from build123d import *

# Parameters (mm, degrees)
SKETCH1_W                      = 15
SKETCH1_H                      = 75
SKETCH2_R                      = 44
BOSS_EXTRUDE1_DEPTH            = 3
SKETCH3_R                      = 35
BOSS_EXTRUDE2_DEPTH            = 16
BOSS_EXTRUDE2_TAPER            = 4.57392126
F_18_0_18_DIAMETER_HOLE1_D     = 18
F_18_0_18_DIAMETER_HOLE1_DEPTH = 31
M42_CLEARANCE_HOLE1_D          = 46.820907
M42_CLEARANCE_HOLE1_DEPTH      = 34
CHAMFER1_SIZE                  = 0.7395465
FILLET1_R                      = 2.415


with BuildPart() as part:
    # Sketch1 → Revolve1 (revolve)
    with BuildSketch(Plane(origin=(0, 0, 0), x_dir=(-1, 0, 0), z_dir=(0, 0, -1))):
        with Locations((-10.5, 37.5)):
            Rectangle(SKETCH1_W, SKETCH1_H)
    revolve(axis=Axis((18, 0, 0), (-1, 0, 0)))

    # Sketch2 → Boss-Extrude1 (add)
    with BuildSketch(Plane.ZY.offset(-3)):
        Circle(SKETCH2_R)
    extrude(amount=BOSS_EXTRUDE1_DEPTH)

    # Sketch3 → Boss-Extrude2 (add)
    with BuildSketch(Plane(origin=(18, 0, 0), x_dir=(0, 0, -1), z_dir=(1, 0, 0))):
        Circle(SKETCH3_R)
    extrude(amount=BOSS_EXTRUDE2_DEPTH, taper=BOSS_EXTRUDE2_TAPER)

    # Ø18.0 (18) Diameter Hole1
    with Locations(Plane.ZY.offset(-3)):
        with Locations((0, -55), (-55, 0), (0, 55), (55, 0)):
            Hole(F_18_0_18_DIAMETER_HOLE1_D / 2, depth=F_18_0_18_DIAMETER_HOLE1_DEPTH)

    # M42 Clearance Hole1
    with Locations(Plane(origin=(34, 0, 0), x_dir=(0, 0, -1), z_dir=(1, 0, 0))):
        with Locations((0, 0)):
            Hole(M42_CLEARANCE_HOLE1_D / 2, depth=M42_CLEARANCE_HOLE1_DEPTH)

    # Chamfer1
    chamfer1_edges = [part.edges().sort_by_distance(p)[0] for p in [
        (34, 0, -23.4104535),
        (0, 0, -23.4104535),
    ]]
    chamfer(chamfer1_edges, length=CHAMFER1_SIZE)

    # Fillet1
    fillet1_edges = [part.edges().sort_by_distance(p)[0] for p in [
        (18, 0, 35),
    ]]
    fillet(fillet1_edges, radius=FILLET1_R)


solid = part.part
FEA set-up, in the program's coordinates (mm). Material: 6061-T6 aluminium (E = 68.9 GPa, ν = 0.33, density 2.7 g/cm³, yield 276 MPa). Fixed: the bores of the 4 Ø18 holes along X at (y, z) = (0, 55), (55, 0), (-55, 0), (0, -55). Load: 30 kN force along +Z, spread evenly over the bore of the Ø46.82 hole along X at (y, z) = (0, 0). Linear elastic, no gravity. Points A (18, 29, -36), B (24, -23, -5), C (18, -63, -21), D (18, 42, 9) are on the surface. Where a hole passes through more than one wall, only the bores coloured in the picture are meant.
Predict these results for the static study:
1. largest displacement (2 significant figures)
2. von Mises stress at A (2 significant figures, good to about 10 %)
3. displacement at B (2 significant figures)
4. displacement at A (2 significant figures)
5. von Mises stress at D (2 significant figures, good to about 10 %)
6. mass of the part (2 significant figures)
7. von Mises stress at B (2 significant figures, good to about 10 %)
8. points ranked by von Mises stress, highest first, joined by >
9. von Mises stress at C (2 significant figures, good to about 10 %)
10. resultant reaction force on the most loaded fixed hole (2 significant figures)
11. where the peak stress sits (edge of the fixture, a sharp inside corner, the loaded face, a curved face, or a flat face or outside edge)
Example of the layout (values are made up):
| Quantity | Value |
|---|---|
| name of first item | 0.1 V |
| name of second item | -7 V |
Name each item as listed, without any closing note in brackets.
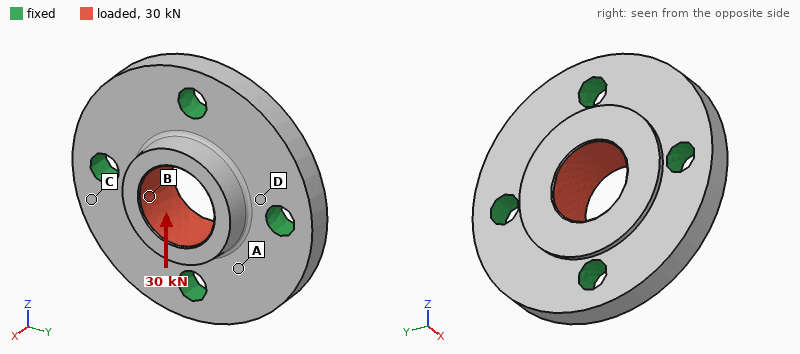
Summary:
| Quantity | Value |
|---|---|
| largest displacement | 14 µm |
| von Mises stress at A | 6.9 MPa |
| displacement at B | 10 µm |
| displacement at A | 4.7 µm |
| von Mises stress at D | 11 MPa |
| mass of the part | 730 g |
| von Mises stress at B | 17 MPa |
| points ranked by von Mises stress, highest first, joined by > | B > D > A > C |
| von Mises stress at C | 3.7 MPa |
| resultant reaction force on the most loaded fixed hole | 9.4 kN |
| where the peak stress sits | a curved face |
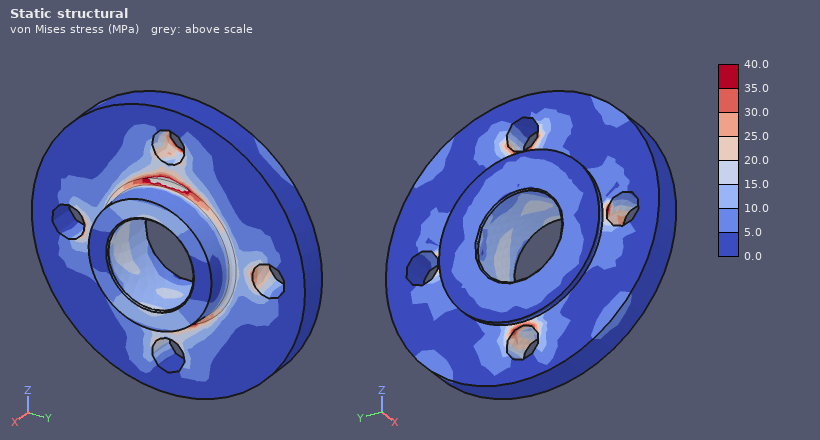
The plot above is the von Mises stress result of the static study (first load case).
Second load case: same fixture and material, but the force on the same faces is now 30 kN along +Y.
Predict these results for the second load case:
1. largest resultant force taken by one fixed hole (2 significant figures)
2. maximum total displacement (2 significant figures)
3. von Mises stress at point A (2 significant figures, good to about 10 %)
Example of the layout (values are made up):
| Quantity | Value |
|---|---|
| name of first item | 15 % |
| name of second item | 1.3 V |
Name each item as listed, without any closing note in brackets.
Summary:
| Quantity | Value |
|---|---|
| largest resultant force taken by one fixed hole | 9.4 kN |
| maximum total displacement | 14 µm |
| von Mises stress at point A | 5.6 MPa |
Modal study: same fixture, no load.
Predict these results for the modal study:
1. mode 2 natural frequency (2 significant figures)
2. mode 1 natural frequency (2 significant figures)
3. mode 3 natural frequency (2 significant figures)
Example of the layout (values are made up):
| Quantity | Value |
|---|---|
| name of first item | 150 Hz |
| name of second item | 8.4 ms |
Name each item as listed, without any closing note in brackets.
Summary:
| Quantity | Value |
|---|---|
| mode 2 natural frequency | 9500 Hz |
| mode 1 natural frequency | 9200 Hz |
| mode 3 natural frequency | 9500 Hz |
